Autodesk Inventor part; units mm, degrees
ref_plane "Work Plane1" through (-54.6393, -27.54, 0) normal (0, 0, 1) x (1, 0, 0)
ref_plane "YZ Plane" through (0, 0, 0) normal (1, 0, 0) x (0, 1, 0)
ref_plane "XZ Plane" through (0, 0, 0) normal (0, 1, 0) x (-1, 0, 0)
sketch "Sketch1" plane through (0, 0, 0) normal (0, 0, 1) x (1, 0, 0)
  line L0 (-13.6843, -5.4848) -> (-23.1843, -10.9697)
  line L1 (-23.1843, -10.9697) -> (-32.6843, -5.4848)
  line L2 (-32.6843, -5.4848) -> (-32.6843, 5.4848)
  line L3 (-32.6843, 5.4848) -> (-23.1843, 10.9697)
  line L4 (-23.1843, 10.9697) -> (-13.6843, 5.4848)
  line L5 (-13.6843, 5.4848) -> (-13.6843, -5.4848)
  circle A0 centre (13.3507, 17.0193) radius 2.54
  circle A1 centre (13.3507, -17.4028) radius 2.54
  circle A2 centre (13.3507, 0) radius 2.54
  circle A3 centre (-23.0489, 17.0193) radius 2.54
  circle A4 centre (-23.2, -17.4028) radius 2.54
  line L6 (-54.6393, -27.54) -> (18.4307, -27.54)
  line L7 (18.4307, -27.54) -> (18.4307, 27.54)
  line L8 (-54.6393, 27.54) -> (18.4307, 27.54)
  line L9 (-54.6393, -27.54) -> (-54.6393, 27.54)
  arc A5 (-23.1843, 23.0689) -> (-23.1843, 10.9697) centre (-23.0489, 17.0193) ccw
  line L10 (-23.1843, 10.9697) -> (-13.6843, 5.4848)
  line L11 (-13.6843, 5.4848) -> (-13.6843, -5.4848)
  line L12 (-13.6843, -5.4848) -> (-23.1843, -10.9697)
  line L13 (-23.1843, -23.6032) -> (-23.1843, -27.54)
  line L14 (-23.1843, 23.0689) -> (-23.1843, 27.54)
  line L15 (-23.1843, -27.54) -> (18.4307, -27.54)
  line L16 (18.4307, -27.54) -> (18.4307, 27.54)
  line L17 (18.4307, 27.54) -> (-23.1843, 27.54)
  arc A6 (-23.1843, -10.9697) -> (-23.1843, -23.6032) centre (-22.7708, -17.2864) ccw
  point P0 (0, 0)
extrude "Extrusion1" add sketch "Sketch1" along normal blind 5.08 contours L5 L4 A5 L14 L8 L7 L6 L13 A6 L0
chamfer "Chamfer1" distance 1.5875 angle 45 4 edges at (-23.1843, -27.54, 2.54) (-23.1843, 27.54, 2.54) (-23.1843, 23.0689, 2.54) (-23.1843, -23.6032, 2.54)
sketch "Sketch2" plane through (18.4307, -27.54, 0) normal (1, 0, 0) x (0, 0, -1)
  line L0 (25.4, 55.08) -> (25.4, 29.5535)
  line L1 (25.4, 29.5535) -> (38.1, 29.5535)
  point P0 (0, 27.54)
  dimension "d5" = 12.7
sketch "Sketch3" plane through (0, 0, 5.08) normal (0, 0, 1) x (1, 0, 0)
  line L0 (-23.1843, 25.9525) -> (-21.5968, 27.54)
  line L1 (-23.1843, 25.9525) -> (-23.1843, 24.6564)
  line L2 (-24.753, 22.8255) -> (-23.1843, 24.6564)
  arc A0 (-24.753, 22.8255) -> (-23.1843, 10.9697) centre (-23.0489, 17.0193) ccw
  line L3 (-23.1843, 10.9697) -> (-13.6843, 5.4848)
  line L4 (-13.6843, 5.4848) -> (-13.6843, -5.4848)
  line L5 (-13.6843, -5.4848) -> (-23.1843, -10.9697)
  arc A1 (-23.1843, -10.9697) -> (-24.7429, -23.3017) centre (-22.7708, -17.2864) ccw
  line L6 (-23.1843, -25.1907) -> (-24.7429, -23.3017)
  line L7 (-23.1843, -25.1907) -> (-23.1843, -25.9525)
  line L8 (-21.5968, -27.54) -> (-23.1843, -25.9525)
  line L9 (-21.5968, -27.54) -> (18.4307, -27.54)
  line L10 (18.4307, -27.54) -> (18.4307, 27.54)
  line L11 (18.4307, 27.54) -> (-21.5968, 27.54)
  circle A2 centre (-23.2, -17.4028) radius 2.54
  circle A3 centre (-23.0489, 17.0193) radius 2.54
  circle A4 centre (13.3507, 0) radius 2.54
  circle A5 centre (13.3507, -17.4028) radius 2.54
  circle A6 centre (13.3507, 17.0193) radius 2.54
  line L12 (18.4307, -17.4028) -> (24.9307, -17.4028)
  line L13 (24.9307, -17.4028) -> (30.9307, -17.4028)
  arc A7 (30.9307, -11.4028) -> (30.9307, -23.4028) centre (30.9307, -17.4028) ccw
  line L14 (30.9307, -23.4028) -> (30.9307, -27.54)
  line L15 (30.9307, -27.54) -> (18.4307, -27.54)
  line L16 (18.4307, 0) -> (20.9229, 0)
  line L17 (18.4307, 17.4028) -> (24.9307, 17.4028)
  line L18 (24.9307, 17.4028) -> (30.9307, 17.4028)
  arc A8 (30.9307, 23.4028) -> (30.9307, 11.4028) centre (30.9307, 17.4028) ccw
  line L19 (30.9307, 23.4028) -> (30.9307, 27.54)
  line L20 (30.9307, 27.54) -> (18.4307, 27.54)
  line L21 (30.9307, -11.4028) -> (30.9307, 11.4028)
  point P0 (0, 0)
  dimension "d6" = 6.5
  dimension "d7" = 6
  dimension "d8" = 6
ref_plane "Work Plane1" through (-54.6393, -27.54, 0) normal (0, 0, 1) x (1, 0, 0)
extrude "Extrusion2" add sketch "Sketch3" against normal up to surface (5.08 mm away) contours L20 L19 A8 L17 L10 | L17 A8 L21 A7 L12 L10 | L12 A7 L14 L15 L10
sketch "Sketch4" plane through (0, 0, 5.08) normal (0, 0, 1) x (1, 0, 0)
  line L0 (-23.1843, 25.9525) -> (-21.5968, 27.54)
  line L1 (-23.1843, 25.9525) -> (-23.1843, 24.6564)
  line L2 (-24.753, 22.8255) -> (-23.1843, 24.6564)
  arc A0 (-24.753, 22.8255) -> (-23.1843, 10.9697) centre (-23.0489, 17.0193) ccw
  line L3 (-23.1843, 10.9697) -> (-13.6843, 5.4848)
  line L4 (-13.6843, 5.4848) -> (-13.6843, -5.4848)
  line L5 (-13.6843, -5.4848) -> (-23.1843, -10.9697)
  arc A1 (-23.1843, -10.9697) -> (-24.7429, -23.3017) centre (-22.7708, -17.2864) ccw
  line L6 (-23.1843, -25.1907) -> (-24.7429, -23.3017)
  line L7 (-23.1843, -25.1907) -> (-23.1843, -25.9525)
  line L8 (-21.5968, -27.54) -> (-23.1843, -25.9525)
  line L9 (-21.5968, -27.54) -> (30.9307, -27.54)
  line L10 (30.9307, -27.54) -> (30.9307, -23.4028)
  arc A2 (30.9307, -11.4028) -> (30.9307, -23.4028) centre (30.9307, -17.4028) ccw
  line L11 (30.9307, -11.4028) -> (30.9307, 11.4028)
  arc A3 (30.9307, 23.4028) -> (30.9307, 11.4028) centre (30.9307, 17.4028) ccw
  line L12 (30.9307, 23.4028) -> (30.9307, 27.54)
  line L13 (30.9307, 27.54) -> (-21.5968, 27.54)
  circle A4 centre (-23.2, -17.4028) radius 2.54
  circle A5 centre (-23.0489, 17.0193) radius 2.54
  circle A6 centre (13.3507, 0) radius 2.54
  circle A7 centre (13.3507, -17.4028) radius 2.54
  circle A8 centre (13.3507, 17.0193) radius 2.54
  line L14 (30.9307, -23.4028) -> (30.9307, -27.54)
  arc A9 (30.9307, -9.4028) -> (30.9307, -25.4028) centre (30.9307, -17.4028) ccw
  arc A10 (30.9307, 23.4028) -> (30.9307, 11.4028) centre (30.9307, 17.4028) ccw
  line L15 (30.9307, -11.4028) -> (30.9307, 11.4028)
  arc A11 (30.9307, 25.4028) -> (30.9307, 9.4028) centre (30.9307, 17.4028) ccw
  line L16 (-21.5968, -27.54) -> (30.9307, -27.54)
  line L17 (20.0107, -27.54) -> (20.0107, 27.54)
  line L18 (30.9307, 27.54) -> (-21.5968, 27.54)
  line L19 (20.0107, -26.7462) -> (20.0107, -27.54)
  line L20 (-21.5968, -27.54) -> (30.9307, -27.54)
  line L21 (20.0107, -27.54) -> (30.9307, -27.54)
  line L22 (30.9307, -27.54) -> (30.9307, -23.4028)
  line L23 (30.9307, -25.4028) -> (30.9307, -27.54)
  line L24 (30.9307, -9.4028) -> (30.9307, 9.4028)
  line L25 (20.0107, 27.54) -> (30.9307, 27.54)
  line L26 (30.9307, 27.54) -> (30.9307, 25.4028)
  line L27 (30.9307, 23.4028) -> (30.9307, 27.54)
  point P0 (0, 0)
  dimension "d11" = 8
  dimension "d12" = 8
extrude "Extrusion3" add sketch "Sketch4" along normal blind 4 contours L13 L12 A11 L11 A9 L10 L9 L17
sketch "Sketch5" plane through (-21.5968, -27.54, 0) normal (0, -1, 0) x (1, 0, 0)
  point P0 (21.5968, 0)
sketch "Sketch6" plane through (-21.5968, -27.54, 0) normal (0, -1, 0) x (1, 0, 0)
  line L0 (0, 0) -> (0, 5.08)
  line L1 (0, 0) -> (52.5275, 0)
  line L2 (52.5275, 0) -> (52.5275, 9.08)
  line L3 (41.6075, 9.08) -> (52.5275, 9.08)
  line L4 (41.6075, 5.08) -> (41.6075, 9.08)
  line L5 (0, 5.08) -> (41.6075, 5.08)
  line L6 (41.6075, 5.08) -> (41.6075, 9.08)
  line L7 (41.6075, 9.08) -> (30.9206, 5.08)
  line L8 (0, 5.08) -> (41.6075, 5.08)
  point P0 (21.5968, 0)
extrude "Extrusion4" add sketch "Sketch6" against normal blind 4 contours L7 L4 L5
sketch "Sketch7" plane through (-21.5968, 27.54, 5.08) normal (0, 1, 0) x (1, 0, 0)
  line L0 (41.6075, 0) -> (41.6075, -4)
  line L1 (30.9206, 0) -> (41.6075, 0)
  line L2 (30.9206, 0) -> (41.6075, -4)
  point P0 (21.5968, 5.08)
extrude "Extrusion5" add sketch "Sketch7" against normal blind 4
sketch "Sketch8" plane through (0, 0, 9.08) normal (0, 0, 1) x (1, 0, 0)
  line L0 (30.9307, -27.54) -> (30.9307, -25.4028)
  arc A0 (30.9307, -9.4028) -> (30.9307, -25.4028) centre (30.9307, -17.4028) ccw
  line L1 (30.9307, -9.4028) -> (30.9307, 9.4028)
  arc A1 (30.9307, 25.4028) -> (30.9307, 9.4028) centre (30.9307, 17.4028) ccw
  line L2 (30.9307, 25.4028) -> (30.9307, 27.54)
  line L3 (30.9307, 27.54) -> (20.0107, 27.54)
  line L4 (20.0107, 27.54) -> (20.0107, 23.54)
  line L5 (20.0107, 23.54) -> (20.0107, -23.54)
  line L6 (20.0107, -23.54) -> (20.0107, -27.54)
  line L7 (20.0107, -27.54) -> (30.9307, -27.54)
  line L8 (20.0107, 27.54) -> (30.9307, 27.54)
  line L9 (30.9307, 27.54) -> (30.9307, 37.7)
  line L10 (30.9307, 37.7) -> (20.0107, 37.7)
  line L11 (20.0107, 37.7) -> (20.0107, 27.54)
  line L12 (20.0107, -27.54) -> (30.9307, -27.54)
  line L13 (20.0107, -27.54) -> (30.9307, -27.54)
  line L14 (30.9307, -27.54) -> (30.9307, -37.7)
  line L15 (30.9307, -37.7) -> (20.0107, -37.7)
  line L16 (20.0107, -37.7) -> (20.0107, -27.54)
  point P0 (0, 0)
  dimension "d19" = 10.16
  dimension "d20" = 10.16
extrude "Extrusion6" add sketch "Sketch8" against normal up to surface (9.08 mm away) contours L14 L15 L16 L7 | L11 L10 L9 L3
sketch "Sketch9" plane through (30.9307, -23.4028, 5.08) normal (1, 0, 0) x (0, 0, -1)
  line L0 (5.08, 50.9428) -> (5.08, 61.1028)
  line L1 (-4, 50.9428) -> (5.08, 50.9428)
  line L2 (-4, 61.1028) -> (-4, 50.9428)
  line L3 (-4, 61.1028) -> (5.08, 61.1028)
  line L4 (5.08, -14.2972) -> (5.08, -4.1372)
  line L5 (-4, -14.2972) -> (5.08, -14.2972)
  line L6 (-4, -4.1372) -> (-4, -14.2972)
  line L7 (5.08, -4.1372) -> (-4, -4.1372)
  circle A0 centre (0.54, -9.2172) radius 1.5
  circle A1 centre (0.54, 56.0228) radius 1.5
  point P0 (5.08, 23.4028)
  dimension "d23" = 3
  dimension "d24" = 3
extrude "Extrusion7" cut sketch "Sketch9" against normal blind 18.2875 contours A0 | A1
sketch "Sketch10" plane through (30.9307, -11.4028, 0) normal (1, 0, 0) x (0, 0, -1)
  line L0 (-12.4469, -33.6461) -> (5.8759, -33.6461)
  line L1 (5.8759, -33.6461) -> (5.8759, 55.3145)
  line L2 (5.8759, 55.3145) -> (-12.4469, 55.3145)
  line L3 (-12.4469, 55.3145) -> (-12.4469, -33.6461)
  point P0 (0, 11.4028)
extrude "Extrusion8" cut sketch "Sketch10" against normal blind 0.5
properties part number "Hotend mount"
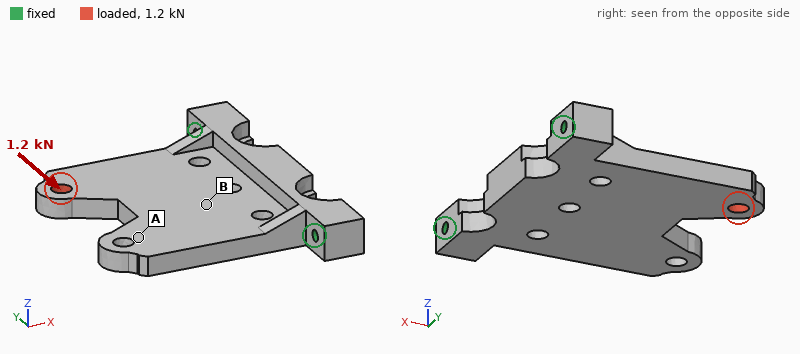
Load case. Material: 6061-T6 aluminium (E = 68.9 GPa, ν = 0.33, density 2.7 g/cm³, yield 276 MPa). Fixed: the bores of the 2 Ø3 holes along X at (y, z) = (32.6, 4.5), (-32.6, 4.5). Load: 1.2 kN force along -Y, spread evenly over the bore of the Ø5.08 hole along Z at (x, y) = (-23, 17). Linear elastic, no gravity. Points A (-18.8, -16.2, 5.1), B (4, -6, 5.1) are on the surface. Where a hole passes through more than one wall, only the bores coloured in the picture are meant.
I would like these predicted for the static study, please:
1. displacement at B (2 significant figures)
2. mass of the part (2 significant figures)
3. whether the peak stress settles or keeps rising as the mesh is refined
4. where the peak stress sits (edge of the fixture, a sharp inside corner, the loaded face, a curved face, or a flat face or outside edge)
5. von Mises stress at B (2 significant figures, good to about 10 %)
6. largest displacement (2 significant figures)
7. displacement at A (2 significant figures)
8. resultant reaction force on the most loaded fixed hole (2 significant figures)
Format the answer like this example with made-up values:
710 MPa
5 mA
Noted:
11 µm
47 g
keeps rising
edge of the fixture
16 MPa
54 µm
22 µm
1.2 kN
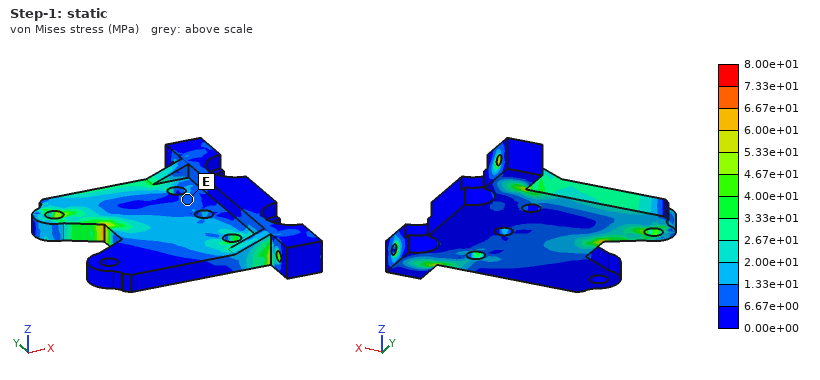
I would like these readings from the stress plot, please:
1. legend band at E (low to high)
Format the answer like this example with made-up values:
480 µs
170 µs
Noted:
6.67e+00 to 1.33e+01 MPa
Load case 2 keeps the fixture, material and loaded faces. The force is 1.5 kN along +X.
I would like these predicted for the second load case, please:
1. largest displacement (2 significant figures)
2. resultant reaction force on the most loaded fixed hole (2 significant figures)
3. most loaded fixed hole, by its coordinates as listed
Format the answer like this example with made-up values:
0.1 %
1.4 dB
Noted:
48 µm
1.3 kN
(32.6, 4.5)
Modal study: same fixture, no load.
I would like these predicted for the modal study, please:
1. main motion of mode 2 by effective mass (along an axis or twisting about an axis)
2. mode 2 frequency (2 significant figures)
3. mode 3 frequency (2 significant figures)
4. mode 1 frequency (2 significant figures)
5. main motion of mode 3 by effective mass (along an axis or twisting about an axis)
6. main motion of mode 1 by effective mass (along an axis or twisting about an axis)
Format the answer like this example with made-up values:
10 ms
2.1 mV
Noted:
twisting about X
3500 Hz
6500 Hz
1500 Hz
along Z
along Z
